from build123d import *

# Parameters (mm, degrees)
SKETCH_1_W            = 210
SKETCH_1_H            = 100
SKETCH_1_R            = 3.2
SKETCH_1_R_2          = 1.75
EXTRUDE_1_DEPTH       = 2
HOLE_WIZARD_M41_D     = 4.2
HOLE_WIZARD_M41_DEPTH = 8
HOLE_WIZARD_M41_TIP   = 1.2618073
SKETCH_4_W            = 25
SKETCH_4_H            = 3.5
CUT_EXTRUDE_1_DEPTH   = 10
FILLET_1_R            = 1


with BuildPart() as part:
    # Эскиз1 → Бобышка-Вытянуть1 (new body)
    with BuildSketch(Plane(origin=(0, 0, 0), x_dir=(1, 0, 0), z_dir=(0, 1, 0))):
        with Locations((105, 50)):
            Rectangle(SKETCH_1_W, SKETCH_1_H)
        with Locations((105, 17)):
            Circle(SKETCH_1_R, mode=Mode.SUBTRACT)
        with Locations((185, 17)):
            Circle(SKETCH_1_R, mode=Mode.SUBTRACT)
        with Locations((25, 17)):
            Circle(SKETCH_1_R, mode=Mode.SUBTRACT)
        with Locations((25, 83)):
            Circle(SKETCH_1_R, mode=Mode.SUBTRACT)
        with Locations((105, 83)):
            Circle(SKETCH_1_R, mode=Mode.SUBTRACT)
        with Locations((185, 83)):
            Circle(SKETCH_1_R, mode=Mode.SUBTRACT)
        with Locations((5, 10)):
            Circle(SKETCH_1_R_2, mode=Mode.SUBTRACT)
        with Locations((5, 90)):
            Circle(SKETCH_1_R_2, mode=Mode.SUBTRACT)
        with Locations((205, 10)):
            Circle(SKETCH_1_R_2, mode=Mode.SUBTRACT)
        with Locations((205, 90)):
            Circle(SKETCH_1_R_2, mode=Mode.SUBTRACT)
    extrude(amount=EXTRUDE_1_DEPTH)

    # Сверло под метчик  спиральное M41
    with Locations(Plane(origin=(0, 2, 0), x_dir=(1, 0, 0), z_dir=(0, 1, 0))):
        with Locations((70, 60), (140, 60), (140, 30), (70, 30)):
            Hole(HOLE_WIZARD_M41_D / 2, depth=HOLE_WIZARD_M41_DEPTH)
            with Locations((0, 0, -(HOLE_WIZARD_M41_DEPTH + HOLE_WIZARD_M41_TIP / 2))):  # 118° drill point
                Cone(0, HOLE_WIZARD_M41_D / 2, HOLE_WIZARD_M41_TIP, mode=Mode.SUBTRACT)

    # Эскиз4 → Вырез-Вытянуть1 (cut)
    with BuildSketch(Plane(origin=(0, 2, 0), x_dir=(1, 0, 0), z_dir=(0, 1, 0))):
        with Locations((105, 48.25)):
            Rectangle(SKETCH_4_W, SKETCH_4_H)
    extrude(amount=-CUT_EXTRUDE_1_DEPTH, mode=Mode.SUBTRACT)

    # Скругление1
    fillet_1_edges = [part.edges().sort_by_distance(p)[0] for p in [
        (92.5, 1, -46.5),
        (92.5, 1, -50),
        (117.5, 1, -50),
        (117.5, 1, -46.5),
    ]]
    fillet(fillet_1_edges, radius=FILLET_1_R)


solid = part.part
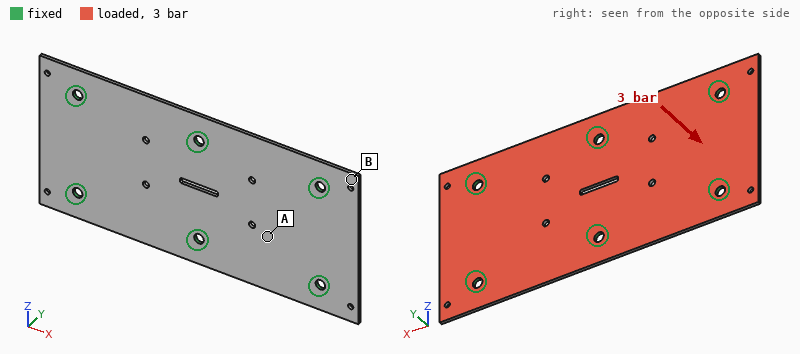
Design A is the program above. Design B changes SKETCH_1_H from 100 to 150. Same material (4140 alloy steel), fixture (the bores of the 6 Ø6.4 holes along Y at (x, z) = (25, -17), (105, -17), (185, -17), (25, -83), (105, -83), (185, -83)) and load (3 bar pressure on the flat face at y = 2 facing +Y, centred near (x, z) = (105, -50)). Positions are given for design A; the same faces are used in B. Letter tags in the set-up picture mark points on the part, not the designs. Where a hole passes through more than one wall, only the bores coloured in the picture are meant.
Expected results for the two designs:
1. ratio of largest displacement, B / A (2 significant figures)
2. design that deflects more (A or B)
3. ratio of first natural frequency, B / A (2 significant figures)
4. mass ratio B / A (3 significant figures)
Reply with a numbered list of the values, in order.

1. 3.6
2. B
3. 0.56
4. 1.51
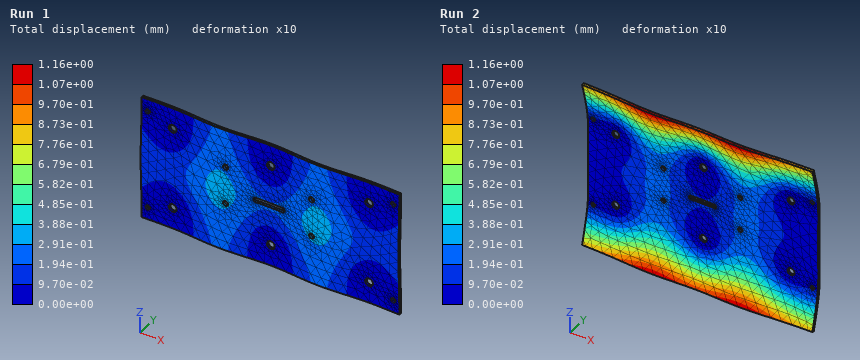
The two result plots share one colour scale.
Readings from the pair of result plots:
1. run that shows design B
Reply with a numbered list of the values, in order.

1. Run 2
